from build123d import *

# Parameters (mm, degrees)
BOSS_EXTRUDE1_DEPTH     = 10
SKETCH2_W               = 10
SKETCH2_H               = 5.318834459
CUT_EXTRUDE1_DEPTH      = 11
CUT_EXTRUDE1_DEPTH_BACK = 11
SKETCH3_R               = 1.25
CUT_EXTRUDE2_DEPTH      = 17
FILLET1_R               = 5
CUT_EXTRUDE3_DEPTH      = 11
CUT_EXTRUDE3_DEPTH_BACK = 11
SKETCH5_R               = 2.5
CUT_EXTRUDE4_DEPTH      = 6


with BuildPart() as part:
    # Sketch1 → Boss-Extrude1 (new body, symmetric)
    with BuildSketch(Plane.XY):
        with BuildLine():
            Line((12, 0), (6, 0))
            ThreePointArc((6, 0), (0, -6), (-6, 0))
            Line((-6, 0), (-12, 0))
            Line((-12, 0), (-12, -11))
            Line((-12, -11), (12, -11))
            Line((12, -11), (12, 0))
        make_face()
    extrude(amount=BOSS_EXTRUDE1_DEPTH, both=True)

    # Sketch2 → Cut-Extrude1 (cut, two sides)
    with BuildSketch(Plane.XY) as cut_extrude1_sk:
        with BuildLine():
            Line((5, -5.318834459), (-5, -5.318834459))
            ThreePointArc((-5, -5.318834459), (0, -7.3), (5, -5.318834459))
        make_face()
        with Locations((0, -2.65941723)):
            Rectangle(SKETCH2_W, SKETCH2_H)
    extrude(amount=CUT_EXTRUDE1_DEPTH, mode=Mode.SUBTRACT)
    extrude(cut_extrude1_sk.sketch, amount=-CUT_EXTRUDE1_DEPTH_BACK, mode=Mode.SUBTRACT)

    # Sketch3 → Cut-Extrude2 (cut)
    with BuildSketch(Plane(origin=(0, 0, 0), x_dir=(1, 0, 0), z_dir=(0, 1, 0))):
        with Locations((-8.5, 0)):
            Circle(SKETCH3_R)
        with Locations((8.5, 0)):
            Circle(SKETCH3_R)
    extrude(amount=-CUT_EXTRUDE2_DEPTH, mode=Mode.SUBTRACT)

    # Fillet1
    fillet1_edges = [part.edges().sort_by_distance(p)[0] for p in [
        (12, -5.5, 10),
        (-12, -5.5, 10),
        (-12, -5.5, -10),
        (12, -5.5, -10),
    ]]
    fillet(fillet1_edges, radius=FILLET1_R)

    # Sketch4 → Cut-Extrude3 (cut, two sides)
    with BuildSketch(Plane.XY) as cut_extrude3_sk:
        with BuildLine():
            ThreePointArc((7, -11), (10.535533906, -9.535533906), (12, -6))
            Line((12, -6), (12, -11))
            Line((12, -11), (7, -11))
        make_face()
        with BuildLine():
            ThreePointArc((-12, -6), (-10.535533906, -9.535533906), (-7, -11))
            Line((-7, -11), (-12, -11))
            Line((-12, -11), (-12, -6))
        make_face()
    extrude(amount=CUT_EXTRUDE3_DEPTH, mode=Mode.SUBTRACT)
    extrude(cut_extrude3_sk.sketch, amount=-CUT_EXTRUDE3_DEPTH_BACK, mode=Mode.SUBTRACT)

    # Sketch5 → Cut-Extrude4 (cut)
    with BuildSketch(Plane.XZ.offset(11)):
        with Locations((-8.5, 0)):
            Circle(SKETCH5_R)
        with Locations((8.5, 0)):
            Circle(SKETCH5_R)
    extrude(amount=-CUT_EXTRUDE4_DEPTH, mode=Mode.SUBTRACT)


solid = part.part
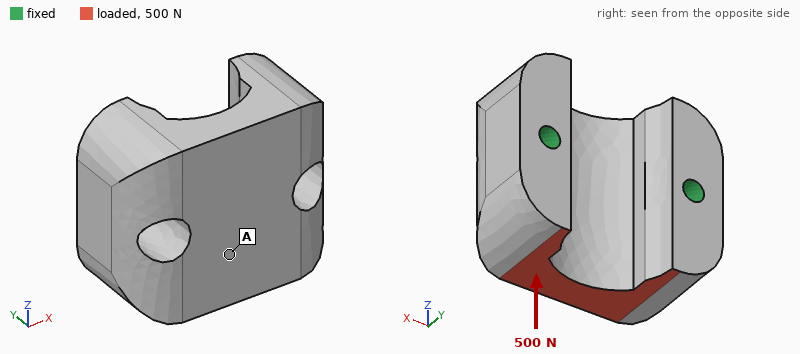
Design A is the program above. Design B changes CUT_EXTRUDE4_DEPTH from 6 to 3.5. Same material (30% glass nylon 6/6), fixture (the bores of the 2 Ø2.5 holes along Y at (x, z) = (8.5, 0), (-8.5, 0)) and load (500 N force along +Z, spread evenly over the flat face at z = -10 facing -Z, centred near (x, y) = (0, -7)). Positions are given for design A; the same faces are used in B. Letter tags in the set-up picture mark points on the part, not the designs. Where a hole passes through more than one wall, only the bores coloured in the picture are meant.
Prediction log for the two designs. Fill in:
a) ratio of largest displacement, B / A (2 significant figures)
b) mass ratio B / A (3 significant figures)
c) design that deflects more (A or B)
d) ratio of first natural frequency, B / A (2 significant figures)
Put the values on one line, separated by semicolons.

0.45; 1.02; A; 1.6
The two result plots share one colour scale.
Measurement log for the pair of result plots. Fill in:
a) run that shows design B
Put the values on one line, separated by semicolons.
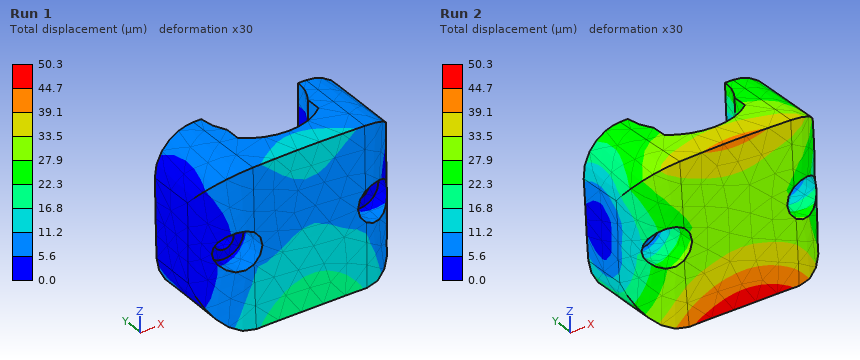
Run 1
